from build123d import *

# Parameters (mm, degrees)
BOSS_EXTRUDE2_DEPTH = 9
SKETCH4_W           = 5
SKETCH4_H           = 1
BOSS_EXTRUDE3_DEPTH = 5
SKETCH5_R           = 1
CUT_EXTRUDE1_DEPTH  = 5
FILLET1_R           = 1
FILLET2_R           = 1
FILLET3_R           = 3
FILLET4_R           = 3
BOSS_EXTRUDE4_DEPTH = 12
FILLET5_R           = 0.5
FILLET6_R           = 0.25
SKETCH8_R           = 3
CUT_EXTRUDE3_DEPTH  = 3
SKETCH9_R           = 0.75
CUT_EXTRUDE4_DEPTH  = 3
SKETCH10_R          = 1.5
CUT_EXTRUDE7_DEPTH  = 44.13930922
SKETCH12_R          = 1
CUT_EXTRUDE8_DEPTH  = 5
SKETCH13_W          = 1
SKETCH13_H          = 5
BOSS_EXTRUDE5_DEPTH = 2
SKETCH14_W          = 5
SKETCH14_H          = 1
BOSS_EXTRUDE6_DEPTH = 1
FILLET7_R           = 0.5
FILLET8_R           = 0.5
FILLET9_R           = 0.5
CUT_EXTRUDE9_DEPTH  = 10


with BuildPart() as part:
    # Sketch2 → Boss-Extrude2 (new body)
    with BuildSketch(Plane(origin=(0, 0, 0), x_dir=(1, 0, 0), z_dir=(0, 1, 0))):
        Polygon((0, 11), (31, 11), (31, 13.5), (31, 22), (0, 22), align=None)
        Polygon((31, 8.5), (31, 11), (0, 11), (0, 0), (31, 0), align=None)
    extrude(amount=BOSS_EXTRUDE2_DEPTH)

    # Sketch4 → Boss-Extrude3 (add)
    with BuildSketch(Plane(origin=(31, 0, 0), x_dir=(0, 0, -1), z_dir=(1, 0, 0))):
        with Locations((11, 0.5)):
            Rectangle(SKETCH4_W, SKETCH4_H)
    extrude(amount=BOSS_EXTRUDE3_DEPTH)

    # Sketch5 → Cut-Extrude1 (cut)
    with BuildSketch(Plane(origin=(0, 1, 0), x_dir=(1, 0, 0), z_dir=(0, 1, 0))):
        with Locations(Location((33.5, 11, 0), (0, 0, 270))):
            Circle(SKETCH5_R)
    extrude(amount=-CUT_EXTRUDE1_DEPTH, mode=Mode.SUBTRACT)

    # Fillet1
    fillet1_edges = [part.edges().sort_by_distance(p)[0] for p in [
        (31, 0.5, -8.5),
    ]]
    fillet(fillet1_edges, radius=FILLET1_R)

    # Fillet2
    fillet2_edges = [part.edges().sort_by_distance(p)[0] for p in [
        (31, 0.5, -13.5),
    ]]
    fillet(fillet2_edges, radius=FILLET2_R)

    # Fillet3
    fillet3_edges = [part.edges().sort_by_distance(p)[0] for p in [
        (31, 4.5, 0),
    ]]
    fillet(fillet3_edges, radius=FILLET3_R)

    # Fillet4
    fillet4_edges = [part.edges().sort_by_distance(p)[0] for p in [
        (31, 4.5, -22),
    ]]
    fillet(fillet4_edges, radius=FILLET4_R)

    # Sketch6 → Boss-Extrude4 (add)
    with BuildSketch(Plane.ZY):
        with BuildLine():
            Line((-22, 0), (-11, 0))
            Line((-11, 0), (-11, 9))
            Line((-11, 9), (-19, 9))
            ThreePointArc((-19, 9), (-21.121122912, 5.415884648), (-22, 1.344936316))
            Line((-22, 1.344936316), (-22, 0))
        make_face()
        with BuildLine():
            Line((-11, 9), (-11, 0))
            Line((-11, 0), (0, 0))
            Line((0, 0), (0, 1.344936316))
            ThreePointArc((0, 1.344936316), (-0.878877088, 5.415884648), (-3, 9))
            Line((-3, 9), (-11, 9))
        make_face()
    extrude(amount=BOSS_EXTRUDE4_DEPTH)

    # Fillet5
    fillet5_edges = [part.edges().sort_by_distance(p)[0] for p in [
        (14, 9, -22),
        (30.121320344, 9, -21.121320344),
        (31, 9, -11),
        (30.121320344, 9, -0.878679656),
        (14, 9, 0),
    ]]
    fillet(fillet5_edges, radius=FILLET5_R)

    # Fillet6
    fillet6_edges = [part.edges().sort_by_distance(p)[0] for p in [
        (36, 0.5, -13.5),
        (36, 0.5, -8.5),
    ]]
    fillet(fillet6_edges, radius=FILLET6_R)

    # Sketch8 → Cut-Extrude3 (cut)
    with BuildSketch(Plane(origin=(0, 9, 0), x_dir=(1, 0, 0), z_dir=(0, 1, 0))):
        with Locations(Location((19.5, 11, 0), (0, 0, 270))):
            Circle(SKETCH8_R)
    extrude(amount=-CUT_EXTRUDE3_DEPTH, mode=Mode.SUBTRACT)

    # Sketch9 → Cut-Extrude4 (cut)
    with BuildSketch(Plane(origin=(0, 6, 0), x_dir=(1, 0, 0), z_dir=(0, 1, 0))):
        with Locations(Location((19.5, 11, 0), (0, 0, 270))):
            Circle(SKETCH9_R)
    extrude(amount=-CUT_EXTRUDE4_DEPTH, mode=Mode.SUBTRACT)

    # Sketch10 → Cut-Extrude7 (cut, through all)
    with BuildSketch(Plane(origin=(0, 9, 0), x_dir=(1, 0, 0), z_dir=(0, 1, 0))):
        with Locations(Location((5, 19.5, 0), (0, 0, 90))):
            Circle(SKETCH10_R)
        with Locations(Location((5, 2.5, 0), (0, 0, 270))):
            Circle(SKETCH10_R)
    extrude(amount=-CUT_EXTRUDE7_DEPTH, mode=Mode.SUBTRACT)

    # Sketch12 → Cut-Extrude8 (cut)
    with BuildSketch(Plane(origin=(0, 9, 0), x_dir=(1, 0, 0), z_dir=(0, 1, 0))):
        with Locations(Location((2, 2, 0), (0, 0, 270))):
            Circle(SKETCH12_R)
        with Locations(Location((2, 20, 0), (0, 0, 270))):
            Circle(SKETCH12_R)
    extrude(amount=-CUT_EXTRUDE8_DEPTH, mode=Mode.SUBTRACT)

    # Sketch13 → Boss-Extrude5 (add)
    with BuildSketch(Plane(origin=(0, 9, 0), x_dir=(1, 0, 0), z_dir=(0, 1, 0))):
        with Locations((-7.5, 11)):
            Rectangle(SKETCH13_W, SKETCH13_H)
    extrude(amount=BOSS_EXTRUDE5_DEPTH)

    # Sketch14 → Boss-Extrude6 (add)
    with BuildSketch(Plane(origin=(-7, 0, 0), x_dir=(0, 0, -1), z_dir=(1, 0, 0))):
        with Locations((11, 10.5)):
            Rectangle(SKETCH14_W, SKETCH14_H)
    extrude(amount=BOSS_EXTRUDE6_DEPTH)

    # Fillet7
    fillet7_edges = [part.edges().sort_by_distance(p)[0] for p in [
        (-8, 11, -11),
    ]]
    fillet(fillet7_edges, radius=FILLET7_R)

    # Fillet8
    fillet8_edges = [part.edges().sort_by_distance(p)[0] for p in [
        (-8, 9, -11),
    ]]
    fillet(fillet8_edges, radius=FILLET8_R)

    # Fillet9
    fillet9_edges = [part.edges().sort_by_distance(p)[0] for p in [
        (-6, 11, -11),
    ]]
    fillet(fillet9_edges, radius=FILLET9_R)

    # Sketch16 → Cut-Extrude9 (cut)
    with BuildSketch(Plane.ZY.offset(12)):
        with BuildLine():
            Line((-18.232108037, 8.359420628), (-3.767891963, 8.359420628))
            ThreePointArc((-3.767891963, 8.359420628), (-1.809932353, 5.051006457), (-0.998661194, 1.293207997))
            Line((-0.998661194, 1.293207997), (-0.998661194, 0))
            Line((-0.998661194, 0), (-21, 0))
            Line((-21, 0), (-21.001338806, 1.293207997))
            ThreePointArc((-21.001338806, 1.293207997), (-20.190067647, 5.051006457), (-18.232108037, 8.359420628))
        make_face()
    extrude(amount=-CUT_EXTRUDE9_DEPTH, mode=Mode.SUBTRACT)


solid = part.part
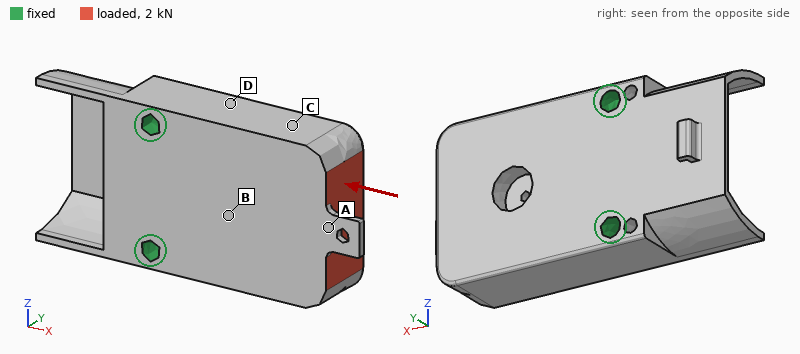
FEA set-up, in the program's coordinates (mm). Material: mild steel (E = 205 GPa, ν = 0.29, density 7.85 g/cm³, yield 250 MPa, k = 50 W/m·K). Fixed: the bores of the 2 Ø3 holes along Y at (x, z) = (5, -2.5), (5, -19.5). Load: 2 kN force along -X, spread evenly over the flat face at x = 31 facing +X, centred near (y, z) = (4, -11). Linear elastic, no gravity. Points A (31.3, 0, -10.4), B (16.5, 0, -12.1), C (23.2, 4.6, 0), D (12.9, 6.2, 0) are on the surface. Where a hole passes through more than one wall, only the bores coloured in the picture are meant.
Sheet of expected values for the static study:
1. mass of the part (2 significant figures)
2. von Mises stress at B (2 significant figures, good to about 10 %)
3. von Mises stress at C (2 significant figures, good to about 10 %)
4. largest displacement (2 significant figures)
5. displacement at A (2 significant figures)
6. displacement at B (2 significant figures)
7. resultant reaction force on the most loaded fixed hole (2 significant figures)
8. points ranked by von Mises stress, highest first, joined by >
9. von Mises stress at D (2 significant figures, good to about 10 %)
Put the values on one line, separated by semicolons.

51 g; 10.0 MPa; 5.6 MPa; 1.8 µm; 1.4 µm; 0.71 µm; 1.0 kN; D > B > C > A; 13 MPa
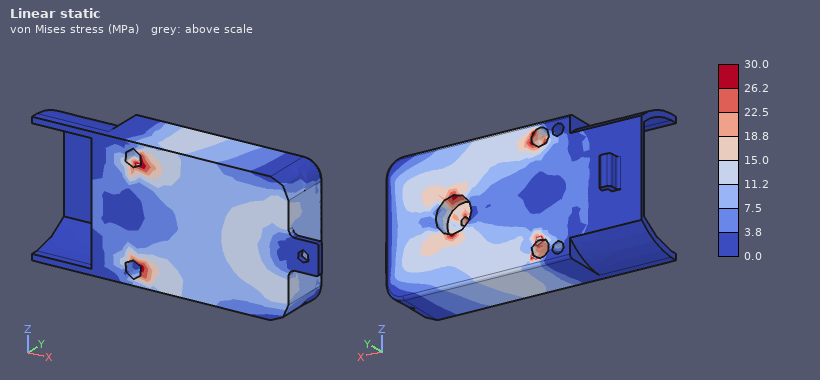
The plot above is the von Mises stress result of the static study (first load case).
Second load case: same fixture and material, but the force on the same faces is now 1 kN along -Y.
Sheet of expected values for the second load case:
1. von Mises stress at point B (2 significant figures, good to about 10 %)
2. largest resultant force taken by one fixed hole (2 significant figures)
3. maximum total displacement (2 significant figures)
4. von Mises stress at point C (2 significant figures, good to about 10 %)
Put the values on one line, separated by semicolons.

49 MPa; 500 N; 35 µm; 18 MPa
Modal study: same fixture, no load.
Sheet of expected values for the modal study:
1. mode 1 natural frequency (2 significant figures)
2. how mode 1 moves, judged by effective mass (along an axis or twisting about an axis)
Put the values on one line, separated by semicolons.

9500 Hz; along Y
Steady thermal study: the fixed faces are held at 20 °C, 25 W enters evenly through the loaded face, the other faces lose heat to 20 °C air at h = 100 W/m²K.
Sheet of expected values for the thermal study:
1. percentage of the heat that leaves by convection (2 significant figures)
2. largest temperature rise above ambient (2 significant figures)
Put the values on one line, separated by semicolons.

22 %; 64 K
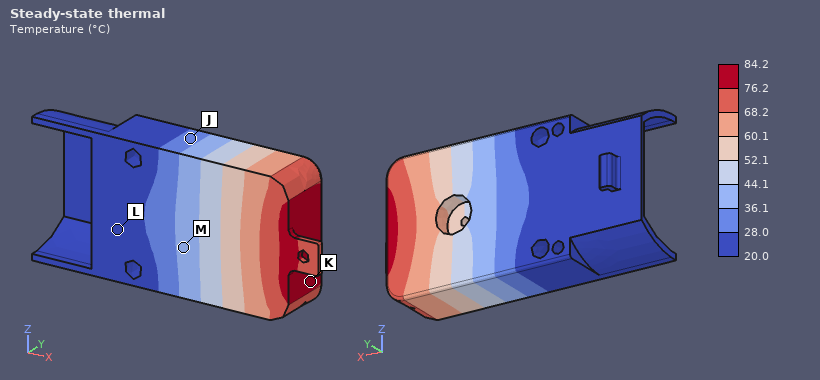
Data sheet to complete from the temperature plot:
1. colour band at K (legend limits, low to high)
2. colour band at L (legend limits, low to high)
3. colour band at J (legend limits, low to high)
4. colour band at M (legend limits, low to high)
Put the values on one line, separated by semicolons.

76.2 to 84.2 °C; 20.0 to 28.0 °C; 28.0 to 36.1 °C; 36.1 to 44.1 °C
